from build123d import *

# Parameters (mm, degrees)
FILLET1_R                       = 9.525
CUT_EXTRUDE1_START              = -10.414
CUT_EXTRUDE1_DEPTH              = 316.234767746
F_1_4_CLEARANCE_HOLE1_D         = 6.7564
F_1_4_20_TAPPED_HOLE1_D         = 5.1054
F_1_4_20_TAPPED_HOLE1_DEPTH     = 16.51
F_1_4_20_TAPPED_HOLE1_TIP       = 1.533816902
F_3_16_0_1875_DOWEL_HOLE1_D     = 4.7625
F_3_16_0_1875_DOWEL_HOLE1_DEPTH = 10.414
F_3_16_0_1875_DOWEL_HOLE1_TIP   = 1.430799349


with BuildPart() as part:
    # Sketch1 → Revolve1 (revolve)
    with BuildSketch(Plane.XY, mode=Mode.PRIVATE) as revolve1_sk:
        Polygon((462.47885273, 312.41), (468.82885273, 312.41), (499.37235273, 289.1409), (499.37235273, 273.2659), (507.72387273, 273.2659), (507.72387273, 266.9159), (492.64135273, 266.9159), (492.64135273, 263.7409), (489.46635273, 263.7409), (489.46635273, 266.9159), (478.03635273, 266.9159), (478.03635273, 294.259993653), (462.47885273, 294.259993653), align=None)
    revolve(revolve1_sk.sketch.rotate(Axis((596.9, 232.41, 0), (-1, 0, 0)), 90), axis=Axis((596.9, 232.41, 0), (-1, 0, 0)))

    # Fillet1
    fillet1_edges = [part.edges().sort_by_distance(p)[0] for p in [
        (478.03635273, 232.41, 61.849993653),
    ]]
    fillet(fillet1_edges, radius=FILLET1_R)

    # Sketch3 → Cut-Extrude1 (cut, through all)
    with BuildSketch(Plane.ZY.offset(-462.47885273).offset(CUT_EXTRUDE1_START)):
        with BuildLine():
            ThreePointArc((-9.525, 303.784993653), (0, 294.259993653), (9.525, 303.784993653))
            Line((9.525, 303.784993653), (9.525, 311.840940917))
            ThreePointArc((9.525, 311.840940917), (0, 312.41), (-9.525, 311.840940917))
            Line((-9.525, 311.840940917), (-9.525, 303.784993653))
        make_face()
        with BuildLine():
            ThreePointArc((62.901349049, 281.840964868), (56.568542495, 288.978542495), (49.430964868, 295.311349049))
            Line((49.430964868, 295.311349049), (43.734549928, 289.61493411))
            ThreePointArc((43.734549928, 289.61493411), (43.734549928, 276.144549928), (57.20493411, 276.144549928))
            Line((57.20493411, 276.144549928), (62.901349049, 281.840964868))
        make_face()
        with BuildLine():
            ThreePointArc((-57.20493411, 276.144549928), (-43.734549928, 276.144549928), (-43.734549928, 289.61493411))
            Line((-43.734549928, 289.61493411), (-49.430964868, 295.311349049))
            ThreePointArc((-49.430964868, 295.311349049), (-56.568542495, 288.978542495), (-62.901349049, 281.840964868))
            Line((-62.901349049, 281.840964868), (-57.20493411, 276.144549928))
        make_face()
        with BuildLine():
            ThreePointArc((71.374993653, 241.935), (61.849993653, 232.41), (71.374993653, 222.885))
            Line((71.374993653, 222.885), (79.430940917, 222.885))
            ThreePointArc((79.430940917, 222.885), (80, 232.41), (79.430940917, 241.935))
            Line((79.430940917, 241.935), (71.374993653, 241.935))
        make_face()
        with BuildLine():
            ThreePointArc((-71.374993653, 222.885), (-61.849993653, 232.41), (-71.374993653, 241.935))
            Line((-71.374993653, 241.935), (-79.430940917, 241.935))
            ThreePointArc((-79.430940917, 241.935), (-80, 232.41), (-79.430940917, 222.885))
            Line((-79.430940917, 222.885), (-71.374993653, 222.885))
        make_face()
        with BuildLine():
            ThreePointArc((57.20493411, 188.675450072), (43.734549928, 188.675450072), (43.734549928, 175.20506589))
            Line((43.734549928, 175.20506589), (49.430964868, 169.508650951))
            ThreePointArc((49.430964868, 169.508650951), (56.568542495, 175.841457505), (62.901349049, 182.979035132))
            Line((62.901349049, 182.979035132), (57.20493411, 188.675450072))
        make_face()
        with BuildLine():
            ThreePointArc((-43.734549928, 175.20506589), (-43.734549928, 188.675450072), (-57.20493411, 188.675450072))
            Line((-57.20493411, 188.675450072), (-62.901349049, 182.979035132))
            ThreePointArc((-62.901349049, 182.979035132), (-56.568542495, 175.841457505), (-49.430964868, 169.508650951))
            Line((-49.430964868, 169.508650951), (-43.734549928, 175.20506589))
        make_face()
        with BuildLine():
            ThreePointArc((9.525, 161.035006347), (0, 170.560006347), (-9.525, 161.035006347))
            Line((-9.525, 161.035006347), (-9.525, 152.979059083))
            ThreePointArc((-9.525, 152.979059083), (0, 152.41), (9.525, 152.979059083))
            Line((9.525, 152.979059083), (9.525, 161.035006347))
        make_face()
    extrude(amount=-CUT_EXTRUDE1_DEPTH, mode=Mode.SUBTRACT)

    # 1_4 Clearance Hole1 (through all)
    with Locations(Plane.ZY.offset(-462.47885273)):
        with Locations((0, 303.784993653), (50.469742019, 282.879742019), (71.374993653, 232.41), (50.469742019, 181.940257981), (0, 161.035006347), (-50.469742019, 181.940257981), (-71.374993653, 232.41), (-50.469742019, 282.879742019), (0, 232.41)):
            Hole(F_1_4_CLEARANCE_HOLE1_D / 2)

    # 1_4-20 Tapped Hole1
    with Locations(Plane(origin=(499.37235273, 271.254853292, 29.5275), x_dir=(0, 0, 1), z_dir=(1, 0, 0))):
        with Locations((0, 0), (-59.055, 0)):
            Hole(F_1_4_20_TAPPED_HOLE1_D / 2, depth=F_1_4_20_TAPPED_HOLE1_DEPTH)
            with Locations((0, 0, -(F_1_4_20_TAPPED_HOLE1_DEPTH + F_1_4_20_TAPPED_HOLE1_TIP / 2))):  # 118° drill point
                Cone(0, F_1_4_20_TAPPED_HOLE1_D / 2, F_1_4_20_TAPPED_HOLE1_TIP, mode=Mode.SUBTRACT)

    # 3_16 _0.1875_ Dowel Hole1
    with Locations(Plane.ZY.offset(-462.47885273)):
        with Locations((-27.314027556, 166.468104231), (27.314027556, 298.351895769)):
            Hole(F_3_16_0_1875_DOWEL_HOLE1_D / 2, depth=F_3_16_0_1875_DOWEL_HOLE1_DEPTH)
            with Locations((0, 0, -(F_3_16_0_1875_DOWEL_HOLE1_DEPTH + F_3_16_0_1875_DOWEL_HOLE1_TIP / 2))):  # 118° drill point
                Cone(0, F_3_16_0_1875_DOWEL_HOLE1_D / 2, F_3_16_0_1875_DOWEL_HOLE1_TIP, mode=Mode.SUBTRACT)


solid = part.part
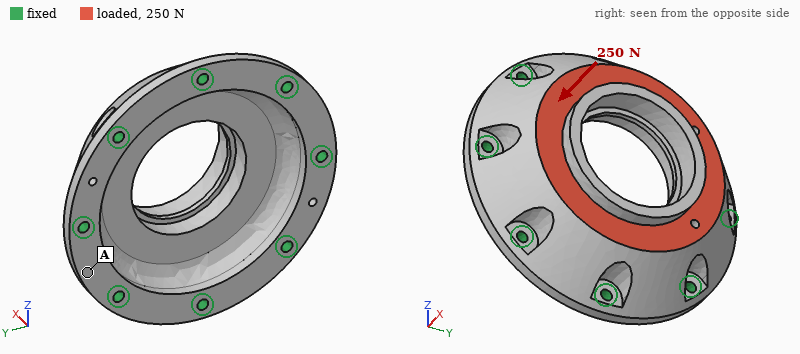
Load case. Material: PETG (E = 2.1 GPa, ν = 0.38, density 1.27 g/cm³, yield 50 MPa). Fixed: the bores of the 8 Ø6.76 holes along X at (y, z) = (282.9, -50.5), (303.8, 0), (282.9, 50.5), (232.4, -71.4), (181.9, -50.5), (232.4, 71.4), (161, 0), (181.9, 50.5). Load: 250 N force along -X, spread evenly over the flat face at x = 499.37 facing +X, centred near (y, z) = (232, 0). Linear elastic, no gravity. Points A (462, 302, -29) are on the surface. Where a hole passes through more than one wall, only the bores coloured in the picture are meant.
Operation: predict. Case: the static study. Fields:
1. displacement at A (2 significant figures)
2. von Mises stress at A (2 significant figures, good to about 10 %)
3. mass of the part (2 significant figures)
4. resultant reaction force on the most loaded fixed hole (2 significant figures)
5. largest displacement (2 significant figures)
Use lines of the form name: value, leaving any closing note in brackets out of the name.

displacement at A: 2.0 µm
von Mises stress at A: 0.082 MPa
mass of the part: 400 g
resultant reaction force on the most loaded fixed hole: 39 N
largest displacement: 6.2 µm
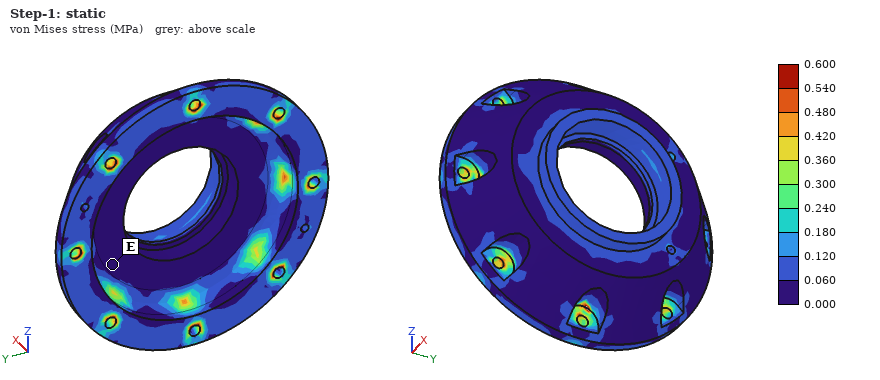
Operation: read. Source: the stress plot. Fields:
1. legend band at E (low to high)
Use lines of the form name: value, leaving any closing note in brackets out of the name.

legend band at E: 0.000 to 0.060 MPa
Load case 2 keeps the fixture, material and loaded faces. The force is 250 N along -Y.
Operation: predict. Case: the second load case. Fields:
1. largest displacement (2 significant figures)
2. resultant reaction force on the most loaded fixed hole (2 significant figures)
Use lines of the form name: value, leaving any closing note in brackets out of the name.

largest displacement: 7.0 µm
resultant reaction force on the most loaded fixed hole: 39 N
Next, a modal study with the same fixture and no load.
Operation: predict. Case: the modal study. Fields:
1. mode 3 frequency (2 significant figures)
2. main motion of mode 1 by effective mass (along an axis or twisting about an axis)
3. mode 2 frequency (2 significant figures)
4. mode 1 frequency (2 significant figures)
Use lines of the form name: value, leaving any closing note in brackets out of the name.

mode 3 frequency: 2300 Hz
main motion of mode 1 by effective mass: along X
mode 2 frequency: 2300 Hz
mode 1 frequency: 2200 Hz
